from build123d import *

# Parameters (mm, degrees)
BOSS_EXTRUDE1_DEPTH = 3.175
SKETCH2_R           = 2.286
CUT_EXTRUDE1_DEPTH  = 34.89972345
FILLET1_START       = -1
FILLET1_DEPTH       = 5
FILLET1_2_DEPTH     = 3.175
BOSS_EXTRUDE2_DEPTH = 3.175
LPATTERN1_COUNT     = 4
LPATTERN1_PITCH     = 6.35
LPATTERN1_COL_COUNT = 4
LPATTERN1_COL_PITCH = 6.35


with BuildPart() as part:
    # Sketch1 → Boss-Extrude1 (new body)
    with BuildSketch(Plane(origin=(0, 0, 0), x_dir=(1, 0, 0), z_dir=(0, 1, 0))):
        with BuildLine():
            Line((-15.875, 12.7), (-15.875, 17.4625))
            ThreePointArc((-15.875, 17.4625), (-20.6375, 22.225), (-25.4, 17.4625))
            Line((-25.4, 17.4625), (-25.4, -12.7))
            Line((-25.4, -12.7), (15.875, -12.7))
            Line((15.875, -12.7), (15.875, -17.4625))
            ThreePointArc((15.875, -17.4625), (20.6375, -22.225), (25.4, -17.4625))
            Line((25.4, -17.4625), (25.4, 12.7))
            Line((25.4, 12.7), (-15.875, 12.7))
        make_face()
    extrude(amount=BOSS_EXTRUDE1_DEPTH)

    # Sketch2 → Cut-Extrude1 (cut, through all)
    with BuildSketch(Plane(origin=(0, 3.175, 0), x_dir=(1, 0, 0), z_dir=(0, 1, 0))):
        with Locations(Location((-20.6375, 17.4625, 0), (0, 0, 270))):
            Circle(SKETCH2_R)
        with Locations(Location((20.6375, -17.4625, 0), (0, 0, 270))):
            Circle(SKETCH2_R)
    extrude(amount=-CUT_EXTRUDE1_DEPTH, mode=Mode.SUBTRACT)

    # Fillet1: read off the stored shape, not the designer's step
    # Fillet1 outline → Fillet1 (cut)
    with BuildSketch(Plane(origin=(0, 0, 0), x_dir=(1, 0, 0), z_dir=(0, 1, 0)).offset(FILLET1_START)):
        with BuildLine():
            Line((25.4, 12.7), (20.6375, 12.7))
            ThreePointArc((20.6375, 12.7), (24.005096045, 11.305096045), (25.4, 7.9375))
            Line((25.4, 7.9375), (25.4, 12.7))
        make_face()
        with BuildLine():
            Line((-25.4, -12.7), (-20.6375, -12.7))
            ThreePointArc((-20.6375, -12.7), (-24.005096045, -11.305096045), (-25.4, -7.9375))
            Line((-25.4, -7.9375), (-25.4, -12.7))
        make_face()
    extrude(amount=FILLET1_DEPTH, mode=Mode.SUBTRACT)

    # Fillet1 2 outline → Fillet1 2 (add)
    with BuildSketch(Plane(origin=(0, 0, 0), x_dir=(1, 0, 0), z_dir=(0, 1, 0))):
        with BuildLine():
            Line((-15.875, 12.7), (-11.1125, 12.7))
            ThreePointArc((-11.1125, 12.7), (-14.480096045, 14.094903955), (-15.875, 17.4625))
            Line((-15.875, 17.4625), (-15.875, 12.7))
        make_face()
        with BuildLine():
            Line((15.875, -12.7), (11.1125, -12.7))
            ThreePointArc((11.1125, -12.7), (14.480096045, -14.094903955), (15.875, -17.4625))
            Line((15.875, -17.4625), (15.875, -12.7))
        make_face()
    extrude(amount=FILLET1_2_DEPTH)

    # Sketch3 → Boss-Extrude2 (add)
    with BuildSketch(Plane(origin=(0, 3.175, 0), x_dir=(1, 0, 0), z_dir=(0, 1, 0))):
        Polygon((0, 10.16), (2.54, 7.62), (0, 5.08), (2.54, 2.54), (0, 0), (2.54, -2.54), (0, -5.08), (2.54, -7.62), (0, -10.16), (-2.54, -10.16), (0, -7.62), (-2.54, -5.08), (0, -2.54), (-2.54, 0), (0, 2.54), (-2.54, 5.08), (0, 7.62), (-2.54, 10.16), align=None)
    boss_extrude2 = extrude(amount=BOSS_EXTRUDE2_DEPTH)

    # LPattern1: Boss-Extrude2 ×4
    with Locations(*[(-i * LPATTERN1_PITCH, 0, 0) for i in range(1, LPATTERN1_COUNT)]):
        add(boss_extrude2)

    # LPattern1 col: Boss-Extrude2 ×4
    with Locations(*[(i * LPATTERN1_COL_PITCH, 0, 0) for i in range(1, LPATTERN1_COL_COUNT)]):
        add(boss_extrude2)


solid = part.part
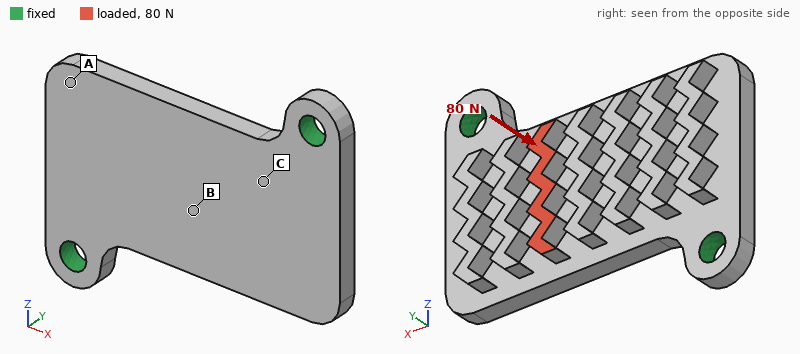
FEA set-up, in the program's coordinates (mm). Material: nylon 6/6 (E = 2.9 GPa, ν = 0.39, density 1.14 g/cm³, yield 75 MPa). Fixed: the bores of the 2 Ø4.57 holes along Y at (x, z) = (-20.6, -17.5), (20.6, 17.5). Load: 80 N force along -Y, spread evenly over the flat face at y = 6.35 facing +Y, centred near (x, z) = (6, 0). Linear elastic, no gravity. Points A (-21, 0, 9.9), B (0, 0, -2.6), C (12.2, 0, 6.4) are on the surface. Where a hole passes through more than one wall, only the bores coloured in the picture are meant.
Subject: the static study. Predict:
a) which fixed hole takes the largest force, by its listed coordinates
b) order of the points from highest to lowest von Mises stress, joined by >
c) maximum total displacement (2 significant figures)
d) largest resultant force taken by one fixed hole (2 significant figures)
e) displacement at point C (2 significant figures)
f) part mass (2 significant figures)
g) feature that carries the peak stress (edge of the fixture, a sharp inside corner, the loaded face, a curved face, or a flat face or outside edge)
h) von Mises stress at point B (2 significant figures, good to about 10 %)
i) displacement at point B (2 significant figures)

(20.6, 17.5)
B > C > A
0.66 mm
51 N
0.25 mm
6.4 g
a flat face or outside edge
7.4 MPa
0.37 mm
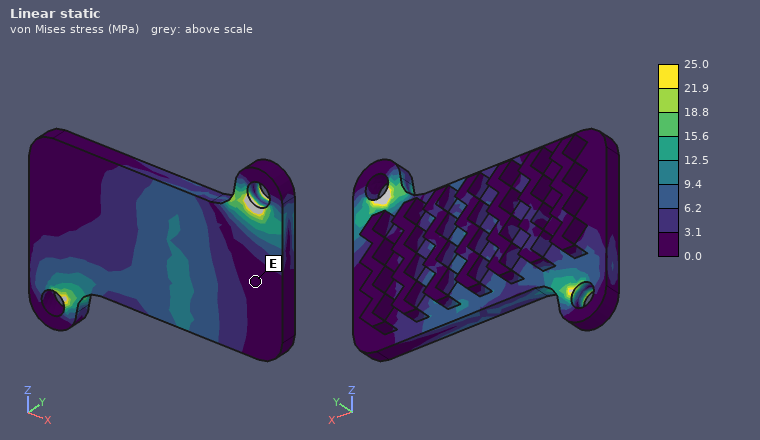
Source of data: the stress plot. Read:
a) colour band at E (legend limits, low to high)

0.0 to 3.1 MPa
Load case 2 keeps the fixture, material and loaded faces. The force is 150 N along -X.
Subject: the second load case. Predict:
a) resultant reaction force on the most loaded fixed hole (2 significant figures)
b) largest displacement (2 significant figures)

80 N
0.49 mm
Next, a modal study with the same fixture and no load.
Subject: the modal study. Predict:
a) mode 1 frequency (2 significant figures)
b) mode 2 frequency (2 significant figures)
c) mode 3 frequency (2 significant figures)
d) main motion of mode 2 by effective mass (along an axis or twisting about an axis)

970 Hz
1200 Hz
2700 Hz
along Y
